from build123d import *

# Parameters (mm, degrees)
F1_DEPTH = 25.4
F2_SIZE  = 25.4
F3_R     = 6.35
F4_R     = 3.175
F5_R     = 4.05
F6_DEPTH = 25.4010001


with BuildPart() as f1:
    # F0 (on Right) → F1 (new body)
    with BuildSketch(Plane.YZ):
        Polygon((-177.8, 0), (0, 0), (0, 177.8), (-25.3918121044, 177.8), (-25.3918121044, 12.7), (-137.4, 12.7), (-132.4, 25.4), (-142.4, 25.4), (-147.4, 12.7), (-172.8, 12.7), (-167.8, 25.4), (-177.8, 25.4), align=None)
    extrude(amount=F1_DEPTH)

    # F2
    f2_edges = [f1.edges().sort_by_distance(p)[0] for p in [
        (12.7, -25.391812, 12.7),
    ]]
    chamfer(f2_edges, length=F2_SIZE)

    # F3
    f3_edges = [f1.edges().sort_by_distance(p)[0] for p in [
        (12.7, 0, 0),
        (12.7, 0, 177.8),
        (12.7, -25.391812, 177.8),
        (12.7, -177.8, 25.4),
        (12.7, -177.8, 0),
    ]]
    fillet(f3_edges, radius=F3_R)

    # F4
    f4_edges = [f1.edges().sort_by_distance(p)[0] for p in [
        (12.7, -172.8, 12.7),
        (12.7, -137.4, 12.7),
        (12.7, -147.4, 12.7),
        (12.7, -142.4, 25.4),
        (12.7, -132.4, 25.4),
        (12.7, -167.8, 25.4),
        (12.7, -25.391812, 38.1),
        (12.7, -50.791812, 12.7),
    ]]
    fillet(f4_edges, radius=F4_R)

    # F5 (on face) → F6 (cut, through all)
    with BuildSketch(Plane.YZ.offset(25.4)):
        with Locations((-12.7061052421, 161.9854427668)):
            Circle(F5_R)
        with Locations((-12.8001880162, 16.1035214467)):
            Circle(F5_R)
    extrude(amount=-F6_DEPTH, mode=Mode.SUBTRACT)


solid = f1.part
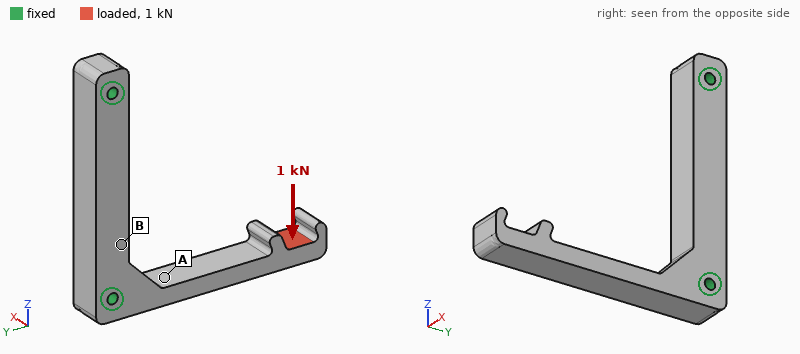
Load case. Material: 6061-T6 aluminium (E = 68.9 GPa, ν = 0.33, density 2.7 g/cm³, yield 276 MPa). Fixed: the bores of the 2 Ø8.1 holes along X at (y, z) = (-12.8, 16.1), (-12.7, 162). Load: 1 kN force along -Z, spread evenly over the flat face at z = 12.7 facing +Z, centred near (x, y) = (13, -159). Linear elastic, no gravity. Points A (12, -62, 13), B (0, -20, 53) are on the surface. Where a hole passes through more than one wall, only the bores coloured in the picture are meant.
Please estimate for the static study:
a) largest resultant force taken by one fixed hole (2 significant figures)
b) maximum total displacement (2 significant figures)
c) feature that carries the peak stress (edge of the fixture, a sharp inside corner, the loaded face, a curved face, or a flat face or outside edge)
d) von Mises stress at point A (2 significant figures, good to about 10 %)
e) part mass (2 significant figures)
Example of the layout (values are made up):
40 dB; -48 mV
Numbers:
730 N; 2.4 mm; a curved face; 140 MPa; 470 g
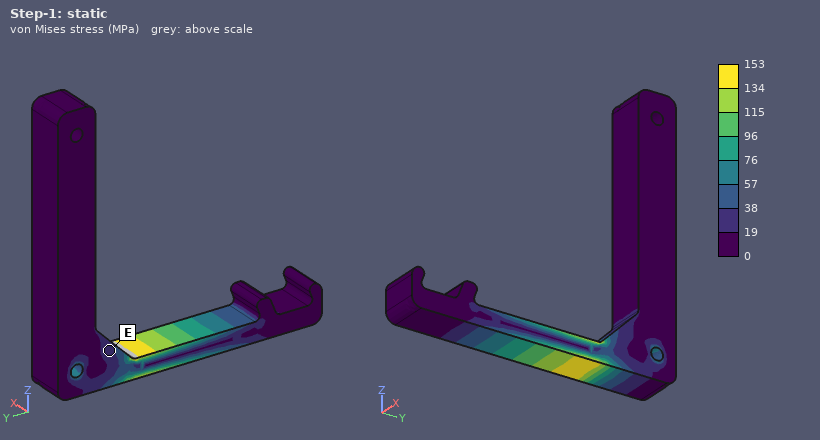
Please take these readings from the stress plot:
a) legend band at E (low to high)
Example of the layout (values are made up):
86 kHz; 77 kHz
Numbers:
19 to 38 MPa
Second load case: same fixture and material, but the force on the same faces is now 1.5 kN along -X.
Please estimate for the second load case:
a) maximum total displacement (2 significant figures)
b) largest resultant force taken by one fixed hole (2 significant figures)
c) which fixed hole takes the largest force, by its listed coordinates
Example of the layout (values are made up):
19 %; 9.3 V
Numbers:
1.3 mm; 1.6 kN; (-12.8, 16.1)
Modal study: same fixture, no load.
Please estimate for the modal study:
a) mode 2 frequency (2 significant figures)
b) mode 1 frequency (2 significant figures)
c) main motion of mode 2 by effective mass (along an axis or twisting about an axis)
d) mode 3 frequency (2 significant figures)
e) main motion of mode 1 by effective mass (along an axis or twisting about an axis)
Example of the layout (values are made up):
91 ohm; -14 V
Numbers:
770 Hz; 470 Hz; along X; 2800 Hz; along Z
